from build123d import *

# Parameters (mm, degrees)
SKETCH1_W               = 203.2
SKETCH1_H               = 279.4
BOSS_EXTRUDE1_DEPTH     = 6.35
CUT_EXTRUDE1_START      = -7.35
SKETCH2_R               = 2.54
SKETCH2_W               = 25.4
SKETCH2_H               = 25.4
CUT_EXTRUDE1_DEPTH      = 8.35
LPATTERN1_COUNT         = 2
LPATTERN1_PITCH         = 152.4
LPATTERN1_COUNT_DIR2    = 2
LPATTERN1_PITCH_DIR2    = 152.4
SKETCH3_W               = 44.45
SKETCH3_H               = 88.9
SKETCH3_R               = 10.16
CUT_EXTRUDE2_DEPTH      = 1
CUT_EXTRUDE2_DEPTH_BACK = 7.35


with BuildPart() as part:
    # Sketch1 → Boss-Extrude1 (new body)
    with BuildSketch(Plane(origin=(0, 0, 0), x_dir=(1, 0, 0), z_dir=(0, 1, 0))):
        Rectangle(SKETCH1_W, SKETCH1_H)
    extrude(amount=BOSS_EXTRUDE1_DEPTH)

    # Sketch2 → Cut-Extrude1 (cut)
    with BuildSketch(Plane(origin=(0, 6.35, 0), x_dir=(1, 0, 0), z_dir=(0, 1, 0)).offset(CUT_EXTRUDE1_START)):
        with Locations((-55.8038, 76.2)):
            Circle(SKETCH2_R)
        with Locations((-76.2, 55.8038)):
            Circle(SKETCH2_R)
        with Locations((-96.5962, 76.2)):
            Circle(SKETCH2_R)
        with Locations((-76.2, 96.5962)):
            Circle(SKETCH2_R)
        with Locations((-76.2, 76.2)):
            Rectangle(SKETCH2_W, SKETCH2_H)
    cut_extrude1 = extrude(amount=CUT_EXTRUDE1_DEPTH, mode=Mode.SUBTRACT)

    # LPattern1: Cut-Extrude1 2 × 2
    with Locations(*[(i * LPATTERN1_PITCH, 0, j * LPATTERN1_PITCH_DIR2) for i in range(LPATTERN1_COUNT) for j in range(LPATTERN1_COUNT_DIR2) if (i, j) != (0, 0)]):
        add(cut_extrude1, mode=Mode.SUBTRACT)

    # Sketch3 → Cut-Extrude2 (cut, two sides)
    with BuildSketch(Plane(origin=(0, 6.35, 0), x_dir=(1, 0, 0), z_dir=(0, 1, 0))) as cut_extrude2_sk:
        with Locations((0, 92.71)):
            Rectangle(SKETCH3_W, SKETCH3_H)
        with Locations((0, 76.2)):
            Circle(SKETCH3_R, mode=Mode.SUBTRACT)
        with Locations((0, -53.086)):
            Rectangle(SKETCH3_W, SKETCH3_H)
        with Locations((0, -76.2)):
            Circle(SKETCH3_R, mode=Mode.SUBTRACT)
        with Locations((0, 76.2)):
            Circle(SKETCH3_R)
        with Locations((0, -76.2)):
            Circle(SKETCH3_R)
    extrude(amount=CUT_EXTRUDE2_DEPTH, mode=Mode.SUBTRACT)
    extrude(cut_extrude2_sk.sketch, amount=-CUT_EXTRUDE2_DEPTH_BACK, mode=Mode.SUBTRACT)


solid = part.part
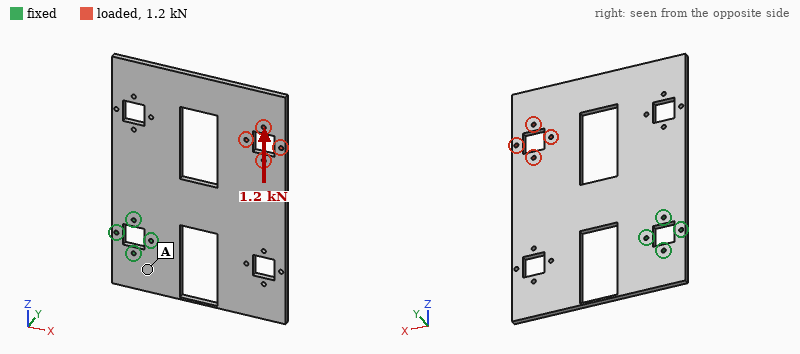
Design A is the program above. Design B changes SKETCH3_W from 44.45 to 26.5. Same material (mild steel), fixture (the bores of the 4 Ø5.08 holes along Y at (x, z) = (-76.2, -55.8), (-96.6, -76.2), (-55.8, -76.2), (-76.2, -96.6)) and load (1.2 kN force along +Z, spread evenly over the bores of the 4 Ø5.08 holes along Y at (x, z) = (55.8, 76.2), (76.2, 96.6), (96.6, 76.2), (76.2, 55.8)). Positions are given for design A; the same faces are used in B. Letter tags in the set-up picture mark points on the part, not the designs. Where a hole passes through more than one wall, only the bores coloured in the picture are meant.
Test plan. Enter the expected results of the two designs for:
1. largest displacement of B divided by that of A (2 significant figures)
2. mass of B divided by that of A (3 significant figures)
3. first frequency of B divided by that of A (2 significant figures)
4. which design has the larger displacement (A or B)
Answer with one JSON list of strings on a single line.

["0.85", "1.07", "1.0", "A"]
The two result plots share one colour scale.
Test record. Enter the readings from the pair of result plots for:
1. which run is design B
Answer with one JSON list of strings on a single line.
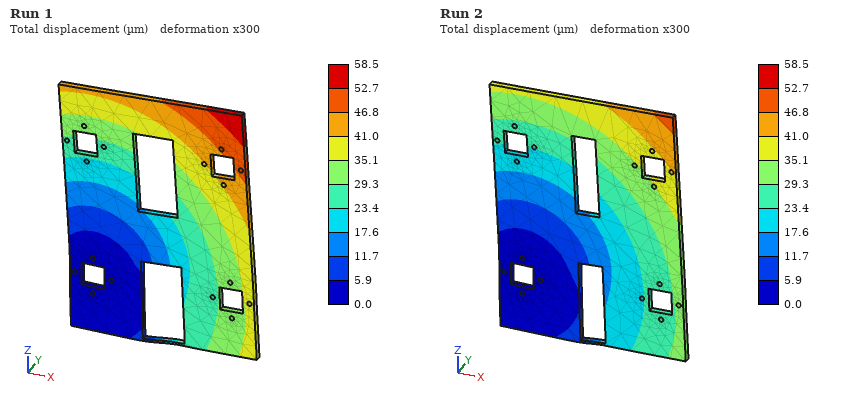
["Run 2"]
